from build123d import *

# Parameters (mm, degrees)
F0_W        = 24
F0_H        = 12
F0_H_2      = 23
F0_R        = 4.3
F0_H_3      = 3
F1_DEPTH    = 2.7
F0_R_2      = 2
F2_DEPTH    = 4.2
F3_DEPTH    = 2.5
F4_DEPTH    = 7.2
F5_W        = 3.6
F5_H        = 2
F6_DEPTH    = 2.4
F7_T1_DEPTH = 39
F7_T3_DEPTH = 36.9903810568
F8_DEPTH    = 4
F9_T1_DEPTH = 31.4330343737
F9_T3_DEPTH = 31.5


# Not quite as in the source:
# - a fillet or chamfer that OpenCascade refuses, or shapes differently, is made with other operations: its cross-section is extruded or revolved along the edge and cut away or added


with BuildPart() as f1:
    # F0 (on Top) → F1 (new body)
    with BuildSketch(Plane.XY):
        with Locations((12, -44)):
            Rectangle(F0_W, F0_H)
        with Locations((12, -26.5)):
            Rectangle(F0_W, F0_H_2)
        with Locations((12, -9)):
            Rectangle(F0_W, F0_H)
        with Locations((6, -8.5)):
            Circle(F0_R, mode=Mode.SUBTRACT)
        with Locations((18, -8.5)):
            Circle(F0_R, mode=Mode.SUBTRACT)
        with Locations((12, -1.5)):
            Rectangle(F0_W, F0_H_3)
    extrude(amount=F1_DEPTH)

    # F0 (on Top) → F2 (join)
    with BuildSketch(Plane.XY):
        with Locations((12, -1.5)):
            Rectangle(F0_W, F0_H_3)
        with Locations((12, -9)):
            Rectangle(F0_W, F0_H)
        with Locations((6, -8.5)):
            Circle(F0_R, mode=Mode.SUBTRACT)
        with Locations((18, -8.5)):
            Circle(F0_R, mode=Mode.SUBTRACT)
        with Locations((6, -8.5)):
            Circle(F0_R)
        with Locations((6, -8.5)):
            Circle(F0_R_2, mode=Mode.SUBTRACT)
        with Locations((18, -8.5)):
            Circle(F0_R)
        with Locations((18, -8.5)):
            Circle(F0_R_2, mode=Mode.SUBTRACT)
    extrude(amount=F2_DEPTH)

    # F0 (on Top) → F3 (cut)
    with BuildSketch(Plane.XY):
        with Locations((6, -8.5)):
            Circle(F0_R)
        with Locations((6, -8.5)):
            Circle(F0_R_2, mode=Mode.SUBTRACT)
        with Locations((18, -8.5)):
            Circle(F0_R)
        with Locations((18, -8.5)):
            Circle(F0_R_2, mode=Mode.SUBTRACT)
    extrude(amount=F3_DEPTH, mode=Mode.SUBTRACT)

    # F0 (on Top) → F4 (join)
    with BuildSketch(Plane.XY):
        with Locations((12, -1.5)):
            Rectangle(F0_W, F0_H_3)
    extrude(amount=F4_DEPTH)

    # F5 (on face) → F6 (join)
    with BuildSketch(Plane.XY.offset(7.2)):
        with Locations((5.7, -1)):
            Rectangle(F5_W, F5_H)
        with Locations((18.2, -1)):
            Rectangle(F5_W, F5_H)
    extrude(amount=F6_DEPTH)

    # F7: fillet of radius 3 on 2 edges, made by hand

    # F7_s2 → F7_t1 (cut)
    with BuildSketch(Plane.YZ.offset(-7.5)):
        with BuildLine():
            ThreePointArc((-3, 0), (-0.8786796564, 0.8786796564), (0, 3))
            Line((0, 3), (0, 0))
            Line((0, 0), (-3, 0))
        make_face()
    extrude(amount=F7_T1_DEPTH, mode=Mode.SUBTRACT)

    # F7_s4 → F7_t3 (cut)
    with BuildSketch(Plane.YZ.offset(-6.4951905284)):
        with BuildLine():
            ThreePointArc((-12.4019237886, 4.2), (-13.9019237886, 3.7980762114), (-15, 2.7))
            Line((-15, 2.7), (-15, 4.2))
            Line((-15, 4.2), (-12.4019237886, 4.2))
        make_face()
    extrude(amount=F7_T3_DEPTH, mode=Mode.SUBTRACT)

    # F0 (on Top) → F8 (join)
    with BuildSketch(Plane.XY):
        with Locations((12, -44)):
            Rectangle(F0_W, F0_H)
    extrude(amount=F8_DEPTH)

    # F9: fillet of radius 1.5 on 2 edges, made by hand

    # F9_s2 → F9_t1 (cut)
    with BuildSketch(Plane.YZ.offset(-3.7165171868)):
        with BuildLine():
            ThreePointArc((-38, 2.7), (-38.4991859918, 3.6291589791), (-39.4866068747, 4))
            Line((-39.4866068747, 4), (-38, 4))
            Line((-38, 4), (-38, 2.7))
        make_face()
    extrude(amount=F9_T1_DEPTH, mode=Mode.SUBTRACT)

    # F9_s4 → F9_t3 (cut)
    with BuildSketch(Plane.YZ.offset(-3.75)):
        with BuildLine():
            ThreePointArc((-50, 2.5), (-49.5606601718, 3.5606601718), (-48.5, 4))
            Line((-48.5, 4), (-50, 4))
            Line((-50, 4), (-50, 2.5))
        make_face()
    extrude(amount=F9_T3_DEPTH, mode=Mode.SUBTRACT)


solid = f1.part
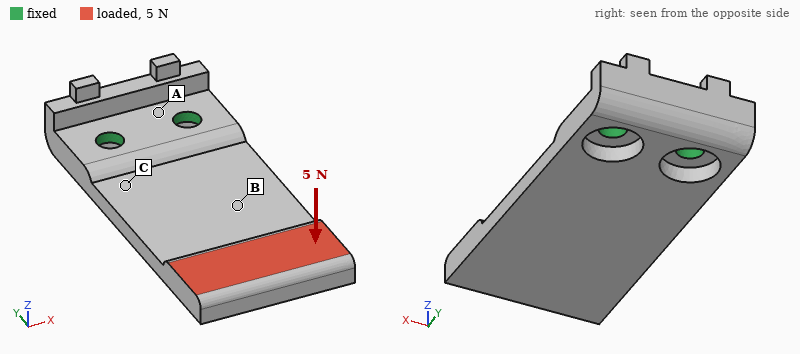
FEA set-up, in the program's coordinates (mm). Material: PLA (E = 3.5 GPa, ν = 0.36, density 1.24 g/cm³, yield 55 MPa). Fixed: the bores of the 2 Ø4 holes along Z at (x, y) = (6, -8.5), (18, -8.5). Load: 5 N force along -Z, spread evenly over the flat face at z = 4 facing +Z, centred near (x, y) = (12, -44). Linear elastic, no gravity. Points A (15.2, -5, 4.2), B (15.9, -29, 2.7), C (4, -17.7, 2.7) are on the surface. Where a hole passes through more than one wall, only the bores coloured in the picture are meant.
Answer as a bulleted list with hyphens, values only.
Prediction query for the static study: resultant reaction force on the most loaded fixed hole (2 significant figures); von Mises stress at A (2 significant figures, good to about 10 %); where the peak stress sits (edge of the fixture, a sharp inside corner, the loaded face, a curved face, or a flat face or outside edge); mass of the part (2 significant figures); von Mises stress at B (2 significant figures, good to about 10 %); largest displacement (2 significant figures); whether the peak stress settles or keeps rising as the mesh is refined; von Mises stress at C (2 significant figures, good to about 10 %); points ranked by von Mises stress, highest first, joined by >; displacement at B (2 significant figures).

- 4.1 N
- 1.0 MPa
- edge of the fixture
- 4.9 g
- 2.4 MPa
- 0.59 mm
- keeps rising
- 4.2 MPa
- C > B > A
- 0.19 mm
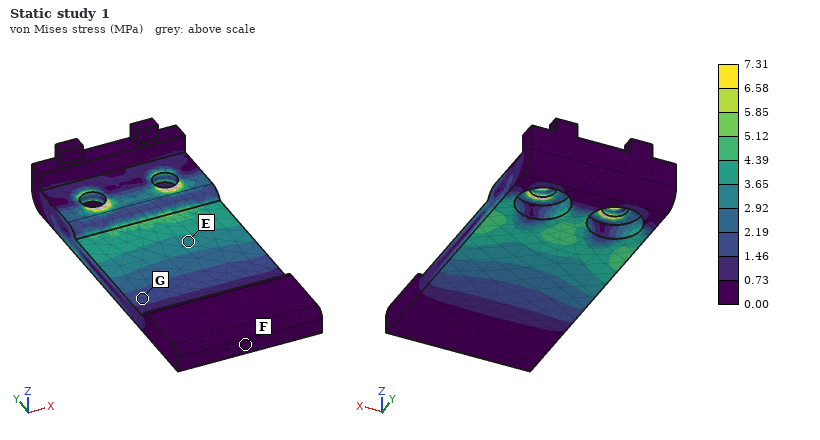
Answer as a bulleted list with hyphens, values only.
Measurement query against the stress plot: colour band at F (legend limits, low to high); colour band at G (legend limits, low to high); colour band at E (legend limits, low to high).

- 0.00 to 0.73 MPa
- 1.46 to 2.19 MPa
- 2.92 to 3.65 MPa
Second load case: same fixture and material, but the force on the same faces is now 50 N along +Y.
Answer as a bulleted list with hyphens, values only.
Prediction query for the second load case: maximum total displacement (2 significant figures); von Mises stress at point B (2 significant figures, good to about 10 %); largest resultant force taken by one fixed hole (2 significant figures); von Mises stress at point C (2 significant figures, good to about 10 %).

- 0.60 mm
- 5.1 MPa
- 26 N
- 5.0 MPa
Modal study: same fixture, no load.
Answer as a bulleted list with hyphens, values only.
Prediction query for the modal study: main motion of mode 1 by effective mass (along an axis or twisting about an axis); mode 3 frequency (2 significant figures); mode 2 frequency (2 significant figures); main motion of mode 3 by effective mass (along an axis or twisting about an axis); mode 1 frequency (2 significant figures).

- along Z
- 2200 Hz
- 1400 Hz
- along X
- 390 Hz
